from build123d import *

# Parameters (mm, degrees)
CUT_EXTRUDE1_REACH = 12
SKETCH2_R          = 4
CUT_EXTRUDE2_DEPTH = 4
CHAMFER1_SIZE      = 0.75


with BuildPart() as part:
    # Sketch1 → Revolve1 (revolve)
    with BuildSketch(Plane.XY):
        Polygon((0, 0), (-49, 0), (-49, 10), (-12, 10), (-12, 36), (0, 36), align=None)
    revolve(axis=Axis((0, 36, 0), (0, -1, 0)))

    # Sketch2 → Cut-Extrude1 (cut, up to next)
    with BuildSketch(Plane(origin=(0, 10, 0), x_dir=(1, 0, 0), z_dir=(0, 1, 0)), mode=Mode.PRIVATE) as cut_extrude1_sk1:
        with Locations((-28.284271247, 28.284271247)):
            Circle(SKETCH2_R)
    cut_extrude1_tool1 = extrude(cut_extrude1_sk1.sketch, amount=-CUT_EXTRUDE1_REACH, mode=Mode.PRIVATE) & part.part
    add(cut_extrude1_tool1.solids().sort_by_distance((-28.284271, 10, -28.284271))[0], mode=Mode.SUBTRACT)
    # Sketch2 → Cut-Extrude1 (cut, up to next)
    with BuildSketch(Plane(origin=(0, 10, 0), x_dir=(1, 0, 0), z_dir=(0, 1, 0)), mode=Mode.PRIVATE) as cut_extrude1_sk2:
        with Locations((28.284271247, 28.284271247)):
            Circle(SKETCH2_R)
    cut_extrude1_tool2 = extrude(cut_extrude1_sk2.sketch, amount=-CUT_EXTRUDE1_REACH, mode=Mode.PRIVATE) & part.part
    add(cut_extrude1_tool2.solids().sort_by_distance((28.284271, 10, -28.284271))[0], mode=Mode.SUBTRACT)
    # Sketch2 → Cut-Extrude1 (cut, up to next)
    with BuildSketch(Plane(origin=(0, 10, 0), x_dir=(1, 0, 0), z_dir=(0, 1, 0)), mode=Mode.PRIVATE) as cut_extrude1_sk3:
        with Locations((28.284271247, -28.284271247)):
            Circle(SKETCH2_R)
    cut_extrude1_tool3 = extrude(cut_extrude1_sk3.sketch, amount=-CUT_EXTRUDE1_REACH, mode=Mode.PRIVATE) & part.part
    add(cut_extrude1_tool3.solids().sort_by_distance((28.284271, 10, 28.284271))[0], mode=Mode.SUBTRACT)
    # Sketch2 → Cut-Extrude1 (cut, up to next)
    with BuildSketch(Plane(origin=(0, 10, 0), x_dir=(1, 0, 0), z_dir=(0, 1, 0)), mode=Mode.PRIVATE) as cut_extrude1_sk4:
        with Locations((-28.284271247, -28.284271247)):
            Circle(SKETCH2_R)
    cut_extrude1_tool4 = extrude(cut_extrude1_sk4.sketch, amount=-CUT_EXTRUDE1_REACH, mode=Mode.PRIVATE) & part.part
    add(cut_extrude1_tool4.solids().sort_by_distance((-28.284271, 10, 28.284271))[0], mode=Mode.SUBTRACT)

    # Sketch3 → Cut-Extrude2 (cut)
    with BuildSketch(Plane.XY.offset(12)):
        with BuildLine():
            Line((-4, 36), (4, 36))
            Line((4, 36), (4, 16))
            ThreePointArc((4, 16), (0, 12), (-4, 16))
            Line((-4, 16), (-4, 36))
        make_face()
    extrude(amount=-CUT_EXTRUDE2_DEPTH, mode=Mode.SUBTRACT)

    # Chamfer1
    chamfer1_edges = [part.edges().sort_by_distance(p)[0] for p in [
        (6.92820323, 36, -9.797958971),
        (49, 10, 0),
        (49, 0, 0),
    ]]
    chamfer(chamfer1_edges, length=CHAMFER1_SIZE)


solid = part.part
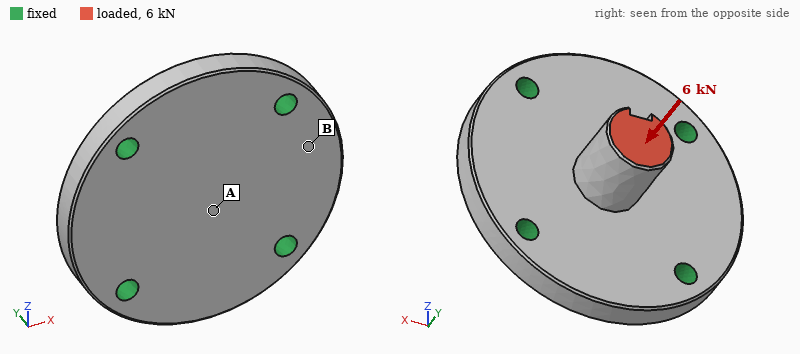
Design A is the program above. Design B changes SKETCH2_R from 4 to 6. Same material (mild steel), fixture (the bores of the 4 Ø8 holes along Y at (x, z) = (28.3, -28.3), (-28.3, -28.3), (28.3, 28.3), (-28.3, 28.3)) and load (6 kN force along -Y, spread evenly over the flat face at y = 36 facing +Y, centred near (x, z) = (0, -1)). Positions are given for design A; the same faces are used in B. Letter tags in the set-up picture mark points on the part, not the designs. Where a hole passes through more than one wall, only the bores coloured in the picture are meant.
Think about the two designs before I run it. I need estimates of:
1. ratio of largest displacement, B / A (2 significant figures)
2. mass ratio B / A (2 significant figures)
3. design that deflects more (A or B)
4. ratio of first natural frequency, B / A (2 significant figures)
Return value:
0.86
0.97
A
1.1
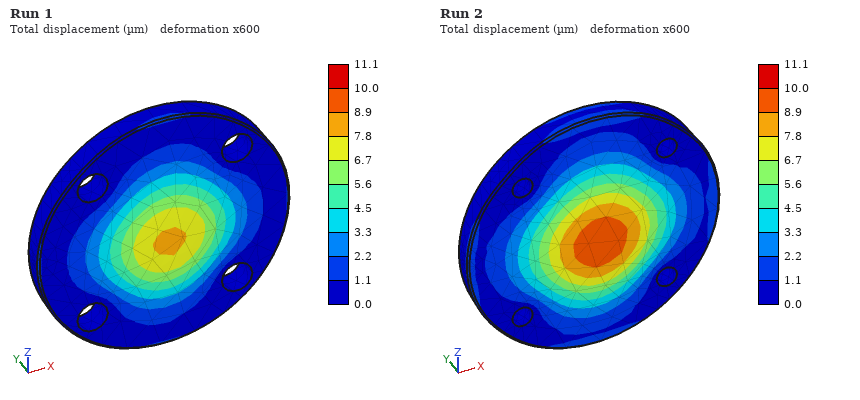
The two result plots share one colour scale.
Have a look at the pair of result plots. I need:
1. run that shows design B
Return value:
Run 1
